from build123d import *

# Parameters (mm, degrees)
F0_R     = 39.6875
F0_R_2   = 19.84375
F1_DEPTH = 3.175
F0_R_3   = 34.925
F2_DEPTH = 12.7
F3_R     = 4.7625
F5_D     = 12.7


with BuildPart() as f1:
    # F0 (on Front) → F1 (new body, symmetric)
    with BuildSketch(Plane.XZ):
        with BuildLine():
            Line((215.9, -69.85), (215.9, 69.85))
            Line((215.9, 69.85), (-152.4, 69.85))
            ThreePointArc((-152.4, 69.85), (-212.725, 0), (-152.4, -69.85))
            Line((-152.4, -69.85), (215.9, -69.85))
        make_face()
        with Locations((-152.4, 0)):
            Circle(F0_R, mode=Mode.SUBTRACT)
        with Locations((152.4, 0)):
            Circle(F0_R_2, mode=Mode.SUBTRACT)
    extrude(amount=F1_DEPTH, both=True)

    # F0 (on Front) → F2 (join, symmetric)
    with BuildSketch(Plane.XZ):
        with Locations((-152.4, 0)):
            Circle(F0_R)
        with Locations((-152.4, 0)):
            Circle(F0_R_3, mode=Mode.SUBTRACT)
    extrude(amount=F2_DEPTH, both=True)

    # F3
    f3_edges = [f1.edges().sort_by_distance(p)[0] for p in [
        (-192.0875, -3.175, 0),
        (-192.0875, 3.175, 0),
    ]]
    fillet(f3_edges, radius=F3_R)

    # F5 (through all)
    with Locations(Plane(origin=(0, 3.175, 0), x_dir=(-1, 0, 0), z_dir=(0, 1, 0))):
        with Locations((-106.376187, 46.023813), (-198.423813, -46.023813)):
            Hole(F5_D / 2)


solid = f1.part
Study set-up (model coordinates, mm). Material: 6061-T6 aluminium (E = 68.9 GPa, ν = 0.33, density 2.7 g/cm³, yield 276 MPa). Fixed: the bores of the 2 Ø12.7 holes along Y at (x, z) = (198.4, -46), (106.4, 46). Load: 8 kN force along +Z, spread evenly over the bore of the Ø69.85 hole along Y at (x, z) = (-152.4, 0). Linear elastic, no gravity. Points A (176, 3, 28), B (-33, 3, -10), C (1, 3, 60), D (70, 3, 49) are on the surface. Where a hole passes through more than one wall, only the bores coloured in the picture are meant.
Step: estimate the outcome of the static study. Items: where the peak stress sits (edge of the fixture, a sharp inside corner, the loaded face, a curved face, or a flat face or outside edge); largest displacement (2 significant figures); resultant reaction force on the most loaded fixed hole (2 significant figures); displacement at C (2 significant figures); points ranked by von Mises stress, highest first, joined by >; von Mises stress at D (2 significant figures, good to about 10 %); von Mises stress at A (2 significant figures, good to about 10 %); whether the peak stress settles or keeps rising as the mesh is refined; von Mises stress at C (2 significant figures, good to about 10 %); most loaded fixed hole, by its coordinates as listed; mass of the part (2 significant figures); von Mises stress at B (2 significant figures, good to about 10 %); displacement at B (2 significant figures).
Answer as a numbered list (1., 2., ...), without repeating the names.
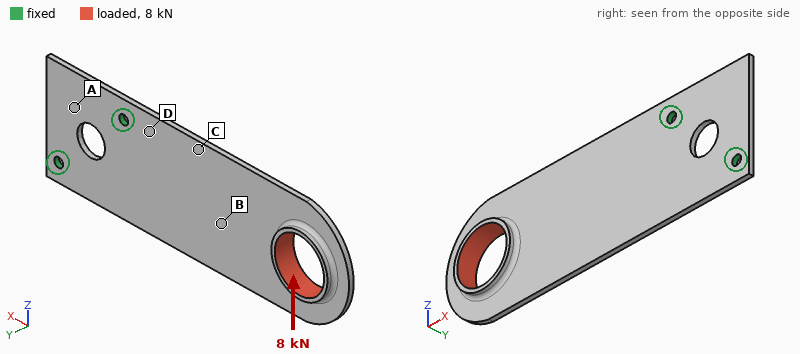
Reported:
1. edge of the fixture
2. 1.1 mm
3. 21 kN
4. 0.29 mm
5. D > C > B > A
6. 67 MPa
7. 9.8 MPa
8. keeps rising
9. 50 MPa
10. (106.4, 46)
11. 960 g
12. 24 MPa
13. 0.38 mm
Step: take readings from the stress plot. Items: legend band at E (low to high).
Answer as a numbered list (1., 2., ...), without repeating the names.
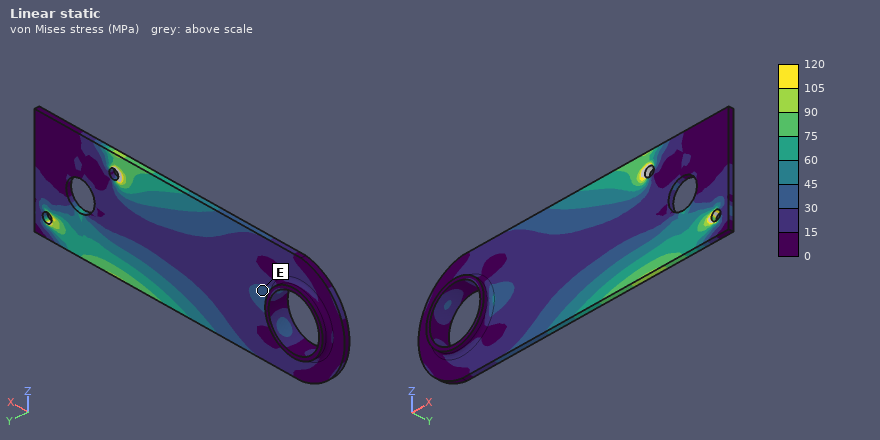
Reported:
1. 30 to 45 MPa
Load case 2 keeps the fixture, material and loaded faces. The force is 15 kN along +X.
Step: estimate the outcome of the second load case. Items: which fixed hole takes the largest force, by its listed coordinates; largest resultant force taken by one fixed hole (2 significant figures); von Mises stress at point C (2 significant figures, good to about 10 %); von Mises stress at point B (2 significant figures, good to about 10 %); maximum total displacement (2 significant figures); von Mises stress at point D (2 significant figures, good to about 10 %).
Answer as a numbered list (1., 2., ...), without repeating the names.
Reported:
1. (106.4, 46)
2. 8.4 kN
3. 17 MPa
4. 16 MPa
5. 0.15 mm
6. 21 MPa
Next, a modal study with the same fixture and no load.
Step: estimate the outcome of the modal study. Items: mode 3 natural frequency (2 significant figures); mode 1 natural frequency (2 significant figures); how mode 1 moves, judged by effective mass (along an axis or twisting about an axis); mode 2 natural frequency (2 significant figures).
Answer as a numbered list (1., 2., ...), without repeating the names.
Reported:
1. 320 Hz
2. 52 Hz
3. along Y
4. 220 Hz
